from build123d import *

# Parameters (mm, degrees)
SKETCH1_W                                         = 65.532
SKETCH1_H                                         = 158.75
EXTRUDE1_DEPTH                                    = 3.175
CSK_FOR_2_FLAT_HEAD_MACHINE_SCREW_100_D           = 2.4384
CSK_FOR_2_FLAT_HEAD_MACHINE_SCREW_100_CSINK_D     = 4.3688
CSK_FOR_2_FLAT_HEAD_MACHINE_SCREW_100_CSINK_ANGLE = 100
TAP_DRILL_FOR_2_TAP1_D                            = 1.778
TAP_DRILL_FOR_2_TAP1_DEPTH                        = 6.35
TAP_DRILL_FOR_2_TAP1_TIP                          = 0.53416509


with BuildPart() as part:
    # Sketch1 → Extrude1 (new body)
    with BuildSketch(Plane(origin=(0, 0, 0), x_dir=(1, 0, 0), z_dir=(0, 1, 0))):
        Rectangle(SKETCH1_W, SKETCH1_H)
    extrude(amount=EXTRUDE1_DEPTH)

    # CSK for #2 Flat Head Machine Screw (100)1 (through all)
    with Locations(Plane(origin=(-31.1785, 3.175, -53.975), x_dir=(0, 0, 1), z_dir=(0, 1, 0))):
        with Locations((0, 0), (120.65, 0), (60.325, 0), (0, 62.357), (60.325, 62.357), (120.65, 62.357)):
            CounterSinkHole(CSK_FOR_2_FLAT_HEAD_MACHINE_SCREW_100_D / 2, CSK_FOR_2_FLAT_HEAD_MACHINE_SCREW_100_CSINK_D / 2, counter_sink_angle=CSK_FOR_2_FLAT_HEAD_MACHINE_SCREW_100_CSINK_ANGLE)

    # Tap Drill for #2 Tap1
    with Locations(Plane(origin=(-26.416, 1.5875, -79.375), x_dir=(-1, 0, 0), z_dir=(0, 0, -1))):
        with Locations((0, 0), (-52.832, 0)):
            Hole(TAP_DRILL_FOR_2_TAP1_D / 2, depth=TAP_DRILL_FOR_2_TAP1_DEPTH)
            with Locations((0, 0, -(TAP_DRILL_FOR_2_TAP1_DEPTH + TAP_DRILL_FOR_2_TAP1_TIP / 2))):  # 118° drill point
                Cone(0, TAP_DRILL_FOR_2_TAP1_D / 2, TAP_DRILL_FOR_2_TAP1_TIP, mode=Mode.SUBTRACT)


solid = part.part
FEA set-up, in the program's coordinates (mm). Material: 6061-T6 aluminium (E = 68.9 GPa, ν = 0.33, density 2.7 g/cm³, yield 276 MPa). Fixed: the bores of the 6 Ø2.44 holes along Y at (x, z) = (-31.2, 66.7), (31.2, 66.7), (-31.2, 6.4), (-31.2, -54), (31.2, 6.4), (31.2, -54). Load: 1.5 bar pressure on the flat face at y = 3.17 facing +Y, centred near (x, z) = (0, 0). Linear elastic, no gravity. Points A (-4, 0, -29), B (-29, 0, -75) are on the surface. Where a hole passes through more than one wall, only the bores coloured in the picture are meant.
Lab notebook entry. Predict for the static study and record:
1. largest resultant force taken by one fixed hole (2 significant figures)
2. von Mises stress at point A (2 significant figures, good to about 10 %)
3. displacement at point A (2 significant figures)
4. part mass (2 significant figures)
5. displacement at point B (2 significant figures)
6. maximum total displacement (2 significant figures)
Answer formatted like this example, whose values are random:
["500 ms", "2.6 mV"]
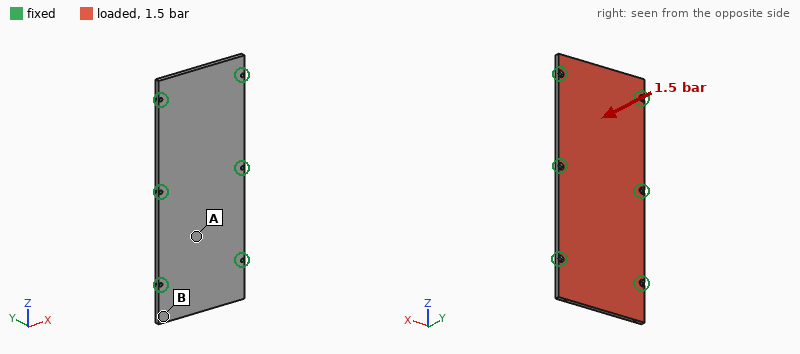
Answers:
["320 N", "19 MPa", "0.091 mm", "89 g", "0.057 mm", "0.14 mm"]
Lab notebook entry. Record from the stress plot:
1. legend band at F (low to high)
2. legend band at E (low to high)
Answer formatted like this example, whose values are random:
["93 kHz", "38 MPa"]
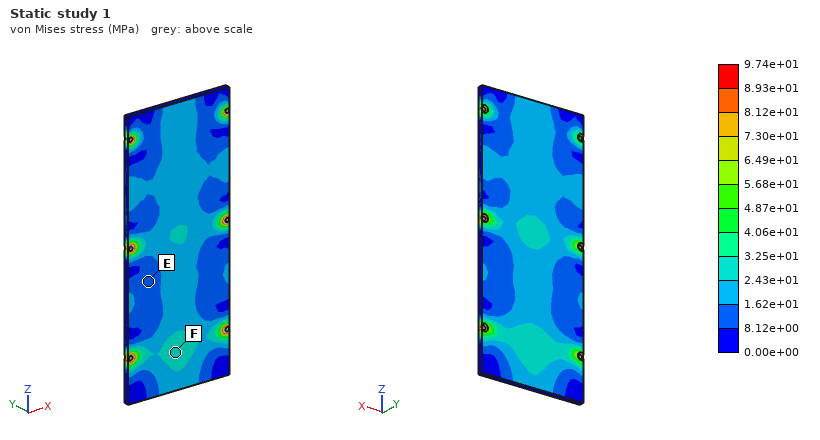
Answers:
["2.43e+01 to 3.25e+01 MPa", "8.12e+00 to 1.62e+01 MPa"]
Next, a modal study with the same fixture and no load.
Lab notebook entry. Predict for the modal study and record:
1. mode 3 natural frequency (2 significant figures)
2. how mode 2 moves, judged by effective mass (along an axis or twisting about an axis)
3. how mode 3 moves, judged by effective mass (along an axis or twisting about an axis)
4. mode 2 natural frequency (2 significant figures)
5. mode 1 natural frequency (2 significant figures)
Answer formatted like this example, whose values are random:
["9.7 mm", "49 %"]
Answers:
["2600 Hz", "along Y", "twisting about X", "2500 Hz", "2200 Hz"]
